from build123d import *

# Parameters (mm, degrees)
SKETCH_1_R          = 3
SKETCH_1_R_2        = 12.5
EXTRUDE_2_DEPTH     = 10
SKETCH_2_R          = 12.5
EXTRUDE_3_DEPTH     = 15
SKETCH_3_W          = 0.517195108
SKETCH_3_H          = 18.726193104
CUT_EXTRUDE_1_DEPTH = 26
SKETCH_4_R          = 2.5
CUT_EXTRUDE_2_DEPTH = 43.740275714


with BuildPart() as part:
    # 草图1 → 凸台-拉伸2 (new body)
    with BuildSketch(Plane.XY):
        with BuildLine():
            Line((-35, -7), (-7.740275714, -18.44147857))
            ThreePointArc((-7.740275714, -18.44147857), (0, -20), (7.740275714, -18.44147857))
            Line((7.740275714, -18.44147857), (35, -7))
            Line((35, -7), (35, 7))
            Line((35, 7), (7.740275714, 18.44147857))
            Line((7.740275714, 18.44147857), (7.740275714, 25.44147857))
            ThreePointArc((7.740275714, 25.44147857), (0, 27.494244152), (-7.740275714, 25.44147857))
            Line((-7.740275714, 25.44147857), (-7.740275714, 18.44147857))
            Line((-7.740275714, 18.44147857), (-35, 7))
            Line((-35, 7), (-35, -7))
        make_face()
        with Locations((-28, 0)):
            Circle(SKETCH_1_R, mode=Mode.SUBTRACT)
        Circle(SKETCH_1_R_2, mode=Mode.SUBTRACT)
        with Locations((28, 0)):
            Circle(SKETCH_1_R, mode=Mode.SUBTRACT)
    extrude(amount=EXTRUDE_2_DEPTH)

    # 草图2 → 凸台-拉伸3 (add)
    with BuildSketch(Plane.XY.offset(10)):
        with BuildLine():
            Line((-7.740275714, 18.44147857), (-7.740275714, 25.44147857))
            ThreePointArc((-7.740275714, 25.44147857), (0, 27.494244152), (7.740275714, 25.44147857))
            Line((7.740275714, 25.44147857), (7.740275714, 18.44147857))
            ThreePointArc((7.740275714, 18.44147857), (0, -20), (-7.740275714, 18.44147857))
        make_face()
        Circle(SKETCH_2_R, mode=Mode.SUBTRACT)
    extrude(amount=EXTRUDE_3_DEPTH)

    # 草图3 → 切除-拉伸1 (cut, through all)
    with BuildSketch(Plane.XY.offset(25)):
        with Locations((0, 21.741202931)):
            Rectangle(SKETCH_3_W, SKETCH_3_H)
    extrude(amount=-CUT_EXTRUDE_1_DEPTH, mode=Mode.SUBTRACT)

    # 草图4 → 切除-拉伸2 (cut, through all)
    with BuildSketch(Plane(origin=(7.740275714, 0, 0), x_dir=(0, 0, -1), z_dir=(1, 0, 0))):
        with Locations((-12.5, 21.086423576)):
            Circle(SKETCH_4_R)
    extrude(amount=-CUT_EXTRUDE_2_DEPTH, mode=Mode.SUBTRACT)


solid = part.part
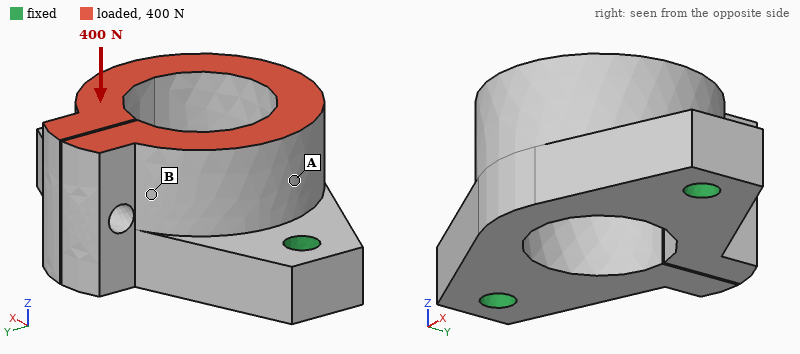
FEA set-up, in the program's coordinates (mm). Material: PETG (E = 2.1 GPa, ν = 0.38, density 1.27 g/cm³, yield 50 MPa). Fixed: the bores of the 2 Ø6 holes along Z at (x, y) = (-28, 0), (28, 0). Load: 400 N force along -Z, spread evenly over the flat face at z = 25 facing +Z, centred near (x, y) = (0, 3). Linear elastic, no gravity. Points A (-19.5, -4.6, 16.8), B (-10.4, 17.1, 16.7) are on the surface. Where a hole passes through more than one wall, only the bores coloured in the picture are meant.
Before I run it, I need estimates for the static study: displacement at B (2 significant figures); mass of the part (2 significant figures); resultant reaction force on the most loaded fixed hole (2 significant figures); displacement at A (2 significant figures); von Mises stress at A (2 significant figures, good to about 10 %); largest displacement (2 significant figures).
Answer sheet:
0.14 mm
36 g
200 N
0.048 mm
2.7 MPa
0.24 mm
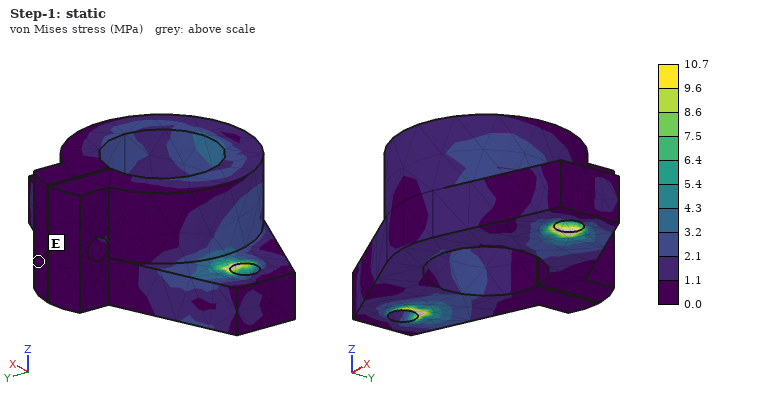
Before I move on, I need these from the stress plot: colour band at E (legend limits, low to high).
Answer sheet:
0.0 to 1.1 MPa
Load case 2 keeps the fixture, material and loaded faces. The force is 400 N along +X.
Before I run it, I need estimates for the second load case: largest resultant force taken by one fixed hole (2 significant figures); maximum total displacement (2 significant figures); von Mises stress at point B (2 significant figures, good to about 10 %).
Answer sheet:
230 N
0.44 mm
2.9 MPa
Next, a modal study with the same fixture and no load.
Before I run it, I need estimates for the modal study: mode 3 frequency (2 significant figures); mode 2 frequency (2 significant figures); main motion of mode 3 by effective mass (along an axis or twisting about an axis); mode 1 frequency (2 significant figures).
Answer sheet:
1500 Hz
1400 Hz
along Y
1400 Hz
